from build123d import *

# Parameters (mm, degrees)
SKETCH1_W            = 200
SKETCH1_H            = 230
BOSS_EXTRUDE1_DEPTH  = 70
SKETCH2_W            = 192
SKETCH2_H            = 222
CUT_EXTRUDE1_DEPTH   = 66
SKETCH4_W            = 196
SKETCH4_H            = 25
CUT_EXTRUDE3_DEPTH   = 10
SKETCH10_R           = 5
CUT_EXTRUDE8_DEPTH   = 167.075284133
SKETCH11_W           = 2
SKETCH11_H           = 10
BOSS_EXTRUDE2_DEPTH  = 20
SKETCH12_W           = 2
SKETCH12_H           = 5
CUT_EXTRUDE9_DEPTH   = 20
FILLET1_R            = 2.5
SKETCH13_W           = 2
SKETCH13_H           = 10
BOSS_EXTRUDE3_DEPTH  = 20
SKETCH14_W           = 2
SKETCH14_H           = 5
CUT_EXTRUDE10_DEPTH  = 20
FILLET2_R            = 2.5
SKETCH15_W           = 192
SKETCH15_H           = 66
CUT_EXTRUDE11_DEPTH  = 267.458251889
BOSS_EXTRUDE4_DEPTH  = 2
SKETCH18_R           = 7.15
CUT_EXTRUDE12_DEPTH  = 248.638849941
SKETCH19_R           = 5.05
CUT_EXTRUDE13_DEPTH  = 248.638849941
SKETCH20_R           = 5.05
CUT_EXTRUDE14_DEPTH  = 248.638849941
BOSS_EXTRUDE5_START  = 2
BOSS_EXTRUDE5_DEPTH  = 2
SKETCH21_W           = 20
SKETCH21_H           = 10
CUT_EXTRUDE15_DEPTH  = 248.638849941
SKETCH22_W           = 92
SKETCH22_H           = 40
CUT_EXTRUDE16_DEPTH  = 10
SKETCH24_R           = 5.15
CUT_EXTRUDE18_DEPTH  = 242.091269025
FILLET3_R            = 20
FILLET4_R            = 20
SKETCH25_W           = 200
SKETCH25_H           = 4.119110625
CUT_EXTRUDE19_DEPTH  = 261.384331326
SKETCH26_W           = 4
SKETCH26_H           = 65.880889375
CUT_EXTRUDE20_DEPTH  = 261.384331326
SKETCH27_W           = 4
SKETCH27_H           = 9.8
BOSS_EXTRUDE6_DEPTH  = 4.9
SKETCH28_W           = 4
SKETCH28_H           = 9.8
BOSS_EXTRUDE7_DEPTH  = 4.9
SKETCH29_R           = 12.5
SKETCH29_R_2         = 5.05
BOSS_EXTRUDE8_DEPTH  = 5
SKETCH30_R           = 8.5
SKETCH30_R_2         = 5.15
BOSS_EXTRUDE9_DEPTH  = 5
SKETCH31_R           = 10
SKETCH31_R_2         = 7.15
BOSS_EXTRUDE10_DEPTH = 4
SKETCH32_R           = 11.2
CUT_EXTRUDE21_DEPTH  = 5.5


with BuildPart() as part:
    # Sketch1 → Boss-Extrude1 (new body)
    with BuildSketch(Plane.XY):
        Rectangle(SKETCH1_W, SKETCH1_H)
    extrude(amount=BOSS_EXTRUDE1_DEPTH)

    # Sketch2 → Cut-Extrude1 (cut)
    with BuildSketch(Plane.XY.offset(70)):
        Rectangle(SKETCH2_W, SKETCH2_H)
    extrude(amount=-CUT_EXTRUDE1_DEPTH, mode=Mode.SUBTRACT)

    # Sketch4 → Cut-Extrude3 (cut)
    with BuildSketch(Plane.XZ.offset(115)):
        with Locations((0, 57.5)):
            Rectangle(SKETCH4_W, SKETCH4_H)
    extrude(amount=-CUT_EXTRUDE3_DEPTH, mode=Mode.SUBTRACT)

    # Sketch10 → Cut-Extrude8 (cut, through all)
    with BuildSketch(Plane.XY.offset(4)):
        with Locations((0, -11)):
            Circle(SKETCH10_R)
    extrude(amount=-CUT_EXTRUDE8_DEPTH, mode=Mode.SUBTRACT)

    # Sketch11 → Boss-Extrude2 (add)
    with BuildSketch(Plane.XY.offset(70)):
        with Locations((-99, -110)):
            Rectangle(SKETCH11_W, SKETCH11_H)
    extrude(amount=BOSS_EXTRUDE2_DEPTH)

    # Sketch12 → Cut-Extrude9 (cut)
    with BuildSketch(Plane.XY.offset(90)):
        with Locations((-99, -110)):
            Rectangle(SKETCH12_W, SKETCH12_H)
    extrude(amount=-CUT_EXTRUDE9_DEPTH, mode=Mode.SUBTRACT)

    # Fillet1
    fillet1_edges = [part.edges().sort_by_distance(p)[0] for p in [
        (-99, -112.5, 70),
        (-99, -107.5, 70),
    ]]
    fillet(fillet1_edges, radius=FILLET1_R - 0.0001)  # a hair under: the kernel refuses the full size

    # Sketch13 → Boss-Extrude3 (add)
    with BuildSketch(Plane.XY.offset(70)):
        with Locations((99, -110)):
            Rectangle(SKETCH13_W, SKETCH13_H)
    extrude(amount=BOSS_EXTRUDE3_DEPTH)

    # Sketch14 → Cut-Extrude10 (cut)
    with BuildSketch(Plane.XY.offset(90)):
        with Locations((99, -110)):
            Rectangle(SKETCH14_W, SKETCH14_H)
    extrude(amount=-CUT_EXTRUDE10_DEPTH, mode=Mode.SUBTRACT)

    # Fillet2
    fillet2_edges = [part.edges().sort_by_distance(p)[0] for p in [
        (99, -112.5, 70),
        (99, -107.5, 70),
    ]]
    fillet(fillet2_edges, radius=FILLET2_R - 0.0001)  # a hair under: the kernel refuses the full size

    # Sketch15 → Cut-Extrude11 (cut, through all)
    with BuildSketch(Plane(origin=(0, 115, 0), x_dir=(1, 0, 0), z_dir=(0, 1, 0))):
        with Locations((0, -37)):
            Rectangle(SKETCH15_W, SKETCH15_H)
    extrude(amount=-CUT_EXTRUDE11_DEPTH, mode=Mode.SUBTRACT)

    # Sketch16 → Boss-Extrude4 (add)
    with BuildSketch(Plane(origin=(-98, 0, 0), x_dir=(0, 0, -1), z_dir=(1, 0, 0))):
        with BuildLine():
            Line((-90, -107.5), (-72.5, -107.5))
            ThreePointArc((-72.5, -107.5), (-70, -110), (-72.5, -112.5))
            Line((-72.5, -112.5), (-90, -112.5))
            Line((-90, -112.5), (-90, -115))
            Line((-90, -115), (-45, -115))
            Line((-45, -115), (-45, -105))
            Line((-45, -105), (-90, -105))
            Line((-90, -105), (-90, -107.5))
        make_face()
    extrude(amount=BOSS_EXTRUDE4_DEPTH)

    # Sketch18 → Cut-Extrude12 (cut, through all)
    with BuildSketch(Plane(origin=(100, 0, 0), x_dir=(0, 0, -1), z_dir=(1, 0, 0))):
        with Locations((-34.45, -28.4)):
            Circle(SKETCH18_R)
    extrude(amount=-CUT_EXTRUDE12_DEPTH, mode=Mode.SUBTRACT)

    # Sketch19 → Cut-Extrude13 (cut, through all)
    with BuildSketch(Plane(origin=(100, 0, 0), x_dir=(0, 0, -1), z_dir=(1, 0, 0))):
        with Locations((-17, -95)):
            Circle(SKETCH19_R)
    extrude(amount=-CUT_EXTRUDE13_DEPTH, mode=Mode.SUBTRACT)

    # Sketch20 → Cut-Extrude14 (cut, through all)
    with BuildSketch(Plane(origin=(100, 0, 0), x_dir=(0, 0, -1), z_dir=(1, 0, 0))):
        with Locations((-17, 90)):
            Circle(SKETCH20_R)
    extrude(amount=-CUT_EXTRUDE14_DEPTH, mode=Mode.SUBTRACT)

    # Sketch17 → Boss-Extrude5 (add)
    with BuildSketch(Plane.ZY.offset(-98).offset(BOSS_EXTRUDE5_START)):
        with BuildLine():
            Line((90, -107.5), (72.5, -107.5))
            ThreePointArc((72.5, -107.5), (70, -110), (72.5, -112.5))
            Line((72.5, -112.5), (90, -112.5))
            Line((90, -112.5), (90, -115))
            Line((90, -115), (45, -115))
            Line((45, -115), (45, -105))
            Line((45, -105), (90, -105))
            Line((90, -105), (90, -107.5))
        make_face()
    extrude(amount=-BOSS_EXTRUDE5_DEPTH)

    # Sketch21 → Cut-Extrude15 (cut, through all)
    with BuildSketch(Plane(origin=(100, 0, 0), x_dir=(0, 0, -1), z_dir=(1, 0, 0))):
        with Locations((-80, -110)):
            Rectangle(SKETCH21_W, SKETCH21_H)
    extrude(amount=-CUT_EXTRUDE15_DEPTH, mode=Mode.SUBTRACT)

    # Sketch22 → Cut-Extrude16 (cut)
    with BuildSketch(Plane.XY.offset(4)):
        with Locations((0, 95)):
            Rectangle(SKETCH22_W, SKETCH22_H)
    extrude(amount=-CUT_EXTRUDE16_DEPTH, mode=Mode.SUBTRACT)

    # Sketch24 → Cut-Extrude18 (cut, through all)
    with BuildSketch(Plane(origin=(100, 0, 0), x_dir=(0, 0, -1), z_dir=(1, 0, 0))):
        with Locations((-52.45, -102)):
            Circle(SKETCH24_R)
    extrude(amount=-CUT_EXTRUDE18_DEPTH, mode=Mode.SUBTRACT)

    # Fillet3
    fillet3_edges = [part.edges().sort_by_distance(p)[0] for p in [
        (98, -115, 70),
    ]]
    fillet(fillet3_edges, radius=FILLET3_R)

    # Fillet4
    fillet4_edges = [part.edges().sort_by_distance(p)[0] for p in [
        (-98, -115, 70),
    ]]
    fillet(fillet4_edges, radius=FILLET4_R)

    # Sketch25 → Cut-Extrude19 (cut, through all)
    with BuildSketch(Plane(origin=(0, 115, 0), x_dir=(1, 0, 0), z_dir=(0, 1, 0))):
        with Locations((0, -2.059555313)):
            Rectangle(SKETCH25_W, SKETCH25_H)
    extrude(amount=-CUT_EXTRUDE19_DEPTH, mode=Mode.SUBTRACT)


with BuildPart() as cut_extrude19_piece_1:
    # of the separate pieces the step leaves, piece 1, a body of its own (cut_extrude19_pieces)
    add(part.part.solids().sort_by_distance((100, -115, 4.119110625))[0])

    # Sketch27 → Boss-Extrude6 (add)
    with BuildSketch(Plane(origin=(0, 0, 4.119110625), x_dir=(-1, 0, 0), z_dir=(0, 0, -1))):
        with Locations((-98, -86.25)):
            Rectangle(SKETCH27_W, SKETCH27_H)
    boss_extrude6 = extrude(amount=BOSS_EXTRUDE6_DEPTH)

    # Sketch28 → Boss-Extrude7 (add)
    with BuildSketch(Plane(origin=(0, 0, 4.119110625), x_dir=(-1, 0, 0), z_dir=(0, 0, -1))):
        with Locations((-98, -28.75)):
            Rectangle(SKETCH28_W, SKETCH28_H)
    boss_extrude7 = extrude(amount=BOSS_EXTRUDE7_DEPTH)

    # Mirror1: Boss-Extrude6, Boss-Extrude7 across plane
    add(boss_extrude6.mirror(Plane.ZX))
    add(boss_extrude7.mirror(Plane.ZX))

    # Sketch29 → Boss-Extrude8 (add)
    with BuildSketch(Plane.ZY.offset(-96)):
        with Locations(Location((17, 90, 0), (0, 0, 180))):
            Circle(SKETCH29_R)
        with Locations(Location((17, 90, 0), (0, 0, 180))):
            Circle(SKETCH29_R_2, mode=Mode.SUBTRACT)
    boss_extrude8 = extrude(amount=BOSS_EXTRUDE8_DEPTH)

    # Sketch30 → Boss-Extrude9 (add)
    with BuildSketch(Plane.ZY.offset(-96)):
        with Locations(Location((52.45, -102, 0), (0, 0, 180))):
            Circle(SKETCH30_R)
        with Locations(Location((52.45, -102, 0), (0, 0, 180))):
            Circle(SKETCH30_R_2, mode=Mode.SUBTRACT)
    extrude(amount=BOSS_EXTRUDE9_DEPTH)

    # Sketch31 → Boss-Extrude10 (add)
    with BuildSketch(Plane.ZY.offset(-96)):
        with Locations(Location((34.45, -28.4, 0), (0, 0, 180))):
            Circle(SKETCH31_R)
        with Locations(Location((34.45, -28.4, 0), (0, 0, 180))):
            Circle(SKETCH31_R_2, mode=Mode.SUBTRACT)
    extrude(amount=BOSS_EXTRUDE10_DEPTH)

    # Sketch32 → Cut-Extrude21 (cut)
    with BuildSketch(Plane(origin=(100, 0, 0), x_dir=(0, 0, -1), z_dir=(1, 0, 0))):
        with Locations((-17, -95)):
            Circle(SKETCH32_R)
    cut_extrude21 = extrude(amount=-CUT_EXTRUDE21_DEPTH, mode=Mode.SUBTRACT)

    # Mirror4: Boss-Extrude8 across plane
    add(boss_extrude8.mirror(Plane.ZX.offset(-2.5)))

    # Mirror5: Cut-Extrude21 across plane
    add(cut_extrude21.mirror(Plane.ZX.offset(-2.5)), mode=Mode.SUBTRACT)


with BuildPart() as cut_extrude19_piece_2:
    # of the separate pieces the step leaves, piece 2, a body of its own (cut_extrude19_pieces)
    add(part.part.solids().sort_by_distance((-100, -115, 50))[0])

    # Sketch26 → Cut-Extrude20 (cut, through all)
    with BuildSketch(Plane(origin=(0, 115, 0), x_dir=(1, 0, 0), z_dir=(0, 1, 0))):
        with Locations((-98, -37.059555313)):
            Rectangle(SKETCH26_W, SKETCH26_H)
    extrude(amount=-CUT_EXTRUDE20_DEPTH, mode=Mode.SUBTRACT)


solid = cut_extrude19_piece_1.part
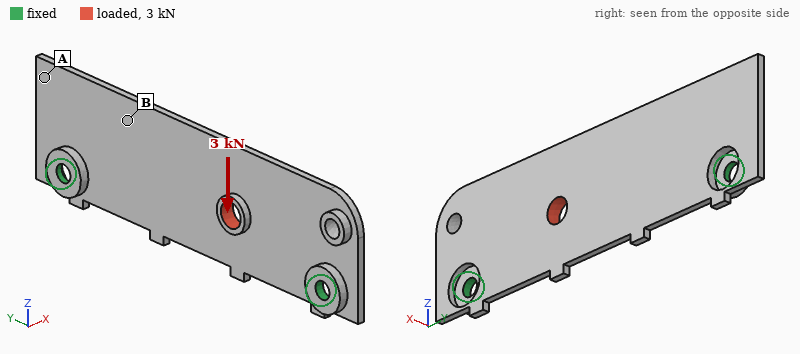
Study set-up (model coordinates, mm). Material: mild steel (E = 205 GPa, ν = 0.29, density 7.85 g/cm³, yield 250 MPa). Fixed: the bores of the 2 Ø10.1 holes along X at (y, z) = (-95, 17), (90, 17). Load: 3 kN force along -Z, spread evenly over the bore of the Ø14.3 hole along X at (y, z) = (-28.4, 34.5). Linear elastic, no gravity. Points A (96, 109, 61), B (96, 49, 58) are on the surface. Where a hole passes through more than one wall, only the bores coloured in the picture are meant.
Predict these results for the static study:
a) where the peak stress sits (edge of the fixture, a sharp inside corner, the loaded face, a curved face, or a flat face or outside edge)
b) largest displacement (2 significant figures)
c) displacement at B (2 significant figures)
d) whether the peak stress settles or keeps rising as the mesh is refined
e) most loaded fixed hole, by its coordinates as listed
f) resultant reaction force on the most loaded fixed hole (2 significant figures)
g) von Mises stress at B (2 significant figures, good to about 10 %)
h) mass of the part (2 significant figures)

edge of the fixture
65 µm
14 µm
keeps rising
(-95, 17)
2.1 kN
16 MPa
490 g
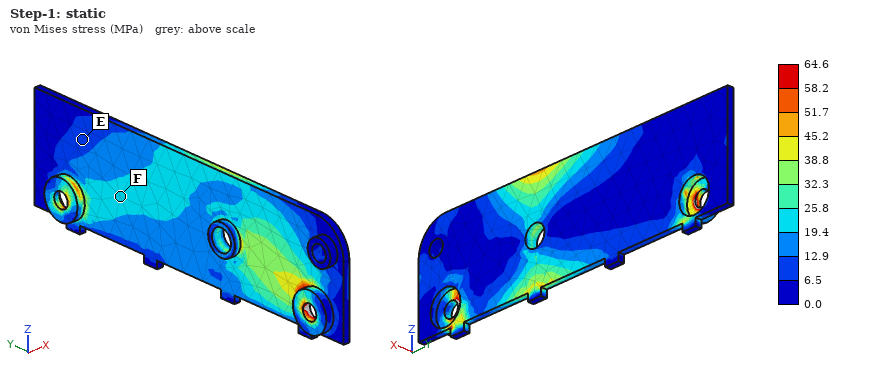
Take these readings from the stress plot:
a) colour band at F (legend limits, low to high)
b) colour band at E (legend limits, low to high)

19.4 to 25.8 MPa
6.5 to 12.9 MPa
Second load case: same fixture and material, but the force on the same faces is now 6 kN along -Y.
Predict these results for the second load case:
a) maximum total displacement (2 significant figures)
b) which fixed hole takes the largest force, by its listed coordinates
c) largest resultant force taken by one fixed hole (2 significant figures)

79 µm
(-95, 17)
3.9 kN
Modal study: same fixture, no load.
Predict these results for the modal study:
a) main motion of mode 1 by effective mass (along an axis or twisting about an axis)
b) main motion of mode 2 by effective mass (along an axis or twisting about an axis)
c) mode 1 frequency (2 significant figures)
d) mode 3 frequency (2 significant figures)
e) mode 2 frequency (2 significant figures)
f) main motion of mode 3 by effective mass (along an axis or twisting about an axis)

along X
twisting about Y
540 Hz
1200 Hz
980 Hz
twisting about Z
